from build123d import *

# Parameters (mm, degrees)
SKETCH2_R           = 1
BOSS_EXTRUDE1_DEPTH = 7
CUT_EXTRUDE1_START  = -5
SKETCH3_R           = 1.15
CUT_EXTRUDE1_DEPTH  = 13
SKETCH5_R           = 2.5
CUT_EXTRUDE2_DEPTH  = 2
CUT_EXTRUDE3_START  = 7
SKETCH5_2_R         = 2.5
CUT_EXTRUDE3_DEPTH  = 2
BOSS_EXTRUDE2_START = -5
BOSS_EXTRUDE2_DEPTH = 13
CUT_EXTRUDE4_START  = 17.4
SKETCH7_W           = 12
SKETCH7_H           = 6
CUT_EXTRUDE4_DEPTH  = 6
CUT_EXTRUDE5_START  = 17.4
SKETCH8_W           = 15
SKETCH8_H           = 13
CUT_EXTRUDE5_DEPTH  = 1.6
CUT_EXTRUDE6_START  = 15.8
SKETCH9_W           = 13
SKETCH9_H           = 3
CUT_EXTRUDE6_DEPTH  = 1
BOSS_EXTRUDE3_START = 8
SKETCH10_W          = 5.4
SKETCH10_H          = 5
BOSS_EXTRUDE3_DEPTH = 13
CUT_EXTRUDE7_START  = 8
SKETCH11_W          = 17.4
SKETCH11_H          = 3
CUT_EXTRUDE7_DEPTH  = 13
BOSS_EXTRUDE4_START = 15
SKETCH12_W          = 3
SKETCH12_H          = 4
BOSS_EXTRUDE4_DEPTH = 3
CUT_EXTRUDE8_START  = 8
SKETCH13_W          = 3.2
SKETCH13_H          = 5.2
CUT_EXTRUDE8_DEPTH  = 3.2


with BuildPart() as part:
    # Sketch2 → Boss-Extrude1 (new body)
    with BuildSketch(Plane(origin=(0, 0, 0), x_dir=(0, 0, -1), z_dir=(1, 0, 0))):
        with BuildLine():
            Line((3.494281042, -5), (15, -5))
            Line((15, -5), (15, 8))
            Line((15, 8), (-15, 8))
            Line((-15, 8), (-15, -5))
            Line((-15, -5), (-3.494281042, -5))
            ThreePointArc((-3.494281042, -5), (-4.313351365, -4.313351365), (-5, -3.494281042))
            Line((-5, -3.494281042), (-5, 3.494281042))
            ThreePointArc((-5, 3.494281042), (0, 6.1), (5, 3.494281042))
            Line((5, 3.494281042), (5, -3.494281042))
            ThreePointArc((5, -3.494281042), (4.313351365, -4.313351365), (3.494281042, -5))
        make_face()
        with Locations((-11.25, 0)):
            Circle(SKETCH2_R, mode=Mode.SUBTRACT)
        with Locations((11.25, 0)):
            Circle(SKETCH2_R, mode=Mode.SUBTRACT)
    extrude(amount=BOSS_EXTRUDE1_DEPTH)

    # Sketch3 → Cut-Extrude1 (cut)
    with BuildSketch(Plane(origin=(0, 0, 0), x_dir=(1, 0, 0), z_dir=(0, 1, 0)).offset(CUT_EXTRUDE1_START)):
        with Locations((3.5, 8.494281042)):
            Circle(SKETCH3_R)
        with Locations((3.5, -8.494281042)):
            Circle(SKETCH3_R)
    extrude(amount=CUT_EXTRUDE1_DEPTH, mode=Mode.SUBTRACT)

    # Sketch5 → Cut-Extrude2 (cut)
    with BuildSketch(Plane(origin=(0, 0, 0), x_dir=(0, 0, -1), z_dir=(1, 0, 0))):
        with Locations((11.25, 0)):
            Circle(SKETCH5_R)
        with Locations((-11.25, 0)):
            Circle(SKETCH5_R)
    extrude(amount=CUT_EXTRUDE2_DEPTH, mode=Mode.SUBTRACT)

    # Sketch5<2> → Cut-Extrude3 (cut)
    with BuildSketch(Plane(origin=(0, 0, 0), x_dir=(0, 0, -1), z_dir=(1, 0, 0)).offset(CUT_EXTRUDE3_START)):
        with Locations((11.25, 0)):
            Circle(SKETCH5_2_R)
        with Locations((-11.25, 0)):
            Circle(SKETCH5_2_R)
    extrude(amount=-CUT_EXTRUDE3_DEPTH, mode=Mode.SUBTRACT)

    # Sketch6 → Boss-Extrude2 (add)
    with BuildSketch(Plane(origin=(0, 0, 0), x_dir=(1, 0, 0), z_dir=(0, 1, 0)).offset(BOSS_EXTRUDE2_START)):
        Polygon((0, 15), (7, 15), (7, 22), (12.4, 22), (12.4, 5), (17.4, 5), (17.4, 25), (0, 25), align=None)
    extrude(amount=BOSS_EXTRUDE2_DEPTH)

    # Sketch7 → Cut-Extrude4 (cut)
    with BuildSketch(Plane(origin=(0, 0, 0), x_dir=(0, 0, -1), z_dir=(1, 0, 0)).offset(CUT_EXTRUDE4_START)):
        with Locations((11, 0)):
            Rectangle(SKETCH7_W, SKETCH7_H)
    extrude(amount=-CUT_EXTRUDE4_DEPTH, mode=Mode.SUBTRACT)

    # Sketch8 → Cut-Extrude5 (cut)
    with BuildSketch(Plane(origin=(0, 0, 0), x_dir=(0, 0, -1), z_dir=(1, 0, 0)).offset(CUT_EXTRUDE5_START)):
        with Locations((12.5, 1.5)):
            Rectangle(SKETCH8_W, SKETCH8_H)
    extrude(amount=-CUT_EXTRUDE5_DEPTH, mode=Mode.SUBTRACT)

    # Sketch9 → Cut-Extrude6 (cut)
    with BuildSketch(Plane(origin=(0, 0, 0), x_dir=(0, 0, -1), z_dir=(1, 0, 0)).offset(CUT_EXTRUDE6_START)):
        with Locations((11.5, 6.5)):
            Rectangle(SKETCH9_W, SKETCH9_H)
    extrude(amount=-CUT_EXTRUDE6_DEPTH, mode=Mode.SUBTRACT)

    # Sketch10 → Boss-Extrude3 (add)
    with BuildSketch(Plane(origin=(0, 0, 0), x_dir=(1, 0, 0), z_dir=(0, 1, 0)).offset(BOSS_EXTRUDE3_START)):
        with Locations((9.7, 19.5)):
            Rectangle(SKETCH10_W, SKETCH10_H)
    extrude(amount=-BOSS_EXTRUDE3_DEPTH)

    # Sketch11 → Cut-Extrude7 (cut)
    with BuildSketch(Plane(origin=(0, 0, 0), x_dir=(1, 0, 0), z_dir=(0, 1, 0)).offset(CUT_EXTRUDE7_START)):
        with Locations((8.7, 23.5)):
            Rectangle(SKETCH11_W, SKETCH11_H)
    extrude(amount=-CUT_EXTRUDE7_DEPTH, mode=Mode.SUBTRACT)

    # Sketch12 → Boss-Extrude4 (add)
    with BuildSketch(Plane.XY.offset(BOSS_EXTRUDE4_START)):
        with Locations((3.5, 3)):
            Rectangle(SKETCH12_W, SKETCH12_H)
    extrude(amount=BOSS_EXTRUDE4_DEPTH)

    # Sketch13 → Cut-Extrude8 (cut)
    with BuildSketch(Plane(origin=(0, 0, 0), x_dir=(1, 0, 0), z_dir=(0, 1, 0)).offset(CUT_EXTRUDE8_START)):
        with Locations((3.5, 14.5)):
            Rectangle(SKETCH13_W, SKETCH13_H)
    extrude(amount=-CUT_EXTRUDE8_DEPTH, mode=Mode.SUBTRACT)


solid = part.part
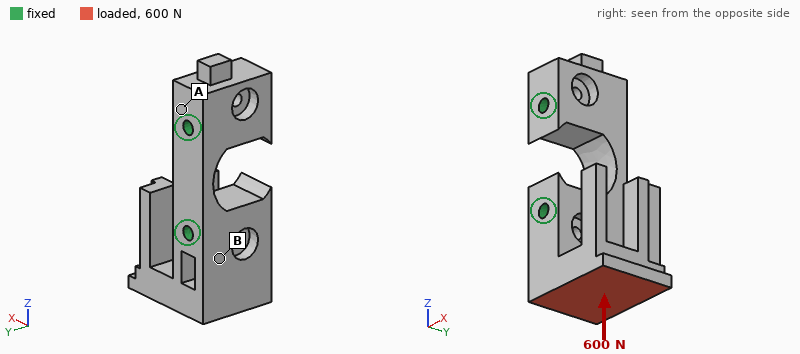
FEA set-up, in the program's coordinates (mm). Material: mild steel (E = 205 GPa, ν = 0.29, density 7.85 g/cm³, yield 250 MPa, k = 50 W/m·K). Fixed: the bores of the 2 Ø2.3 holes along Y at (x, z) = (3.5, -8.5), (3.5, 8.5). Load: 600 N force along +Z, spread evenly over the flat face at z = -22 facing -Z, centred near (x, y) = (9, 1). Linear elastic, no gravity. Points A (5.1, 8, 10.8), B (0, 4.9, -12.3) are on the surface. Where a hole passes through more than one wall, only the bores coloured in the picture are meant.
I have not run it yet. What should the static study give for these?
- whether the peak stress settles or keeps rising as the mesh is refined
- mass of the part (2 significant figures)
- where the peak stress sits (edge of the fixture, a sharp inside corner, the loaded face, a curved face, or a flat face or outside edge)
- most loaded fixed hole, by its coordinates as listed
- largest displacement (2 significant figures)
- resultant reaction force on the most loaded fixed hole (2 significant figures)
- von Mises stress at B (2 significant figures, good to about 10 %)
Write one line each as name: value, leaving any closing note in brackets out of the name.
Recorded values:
whether the peak stress settles or keeps rising as the mesh is refined: keeps rising
mass of the part: 25 g
where the peak stress sits: edge of the fixture
most loaded fixed hole, by its coordinates as listed: (3.5, -8.5)
largest displacement: 16 µm
resultant reaction force on the most loaded fixed hole: 590 N
von Mises stress at B: 36 MPa
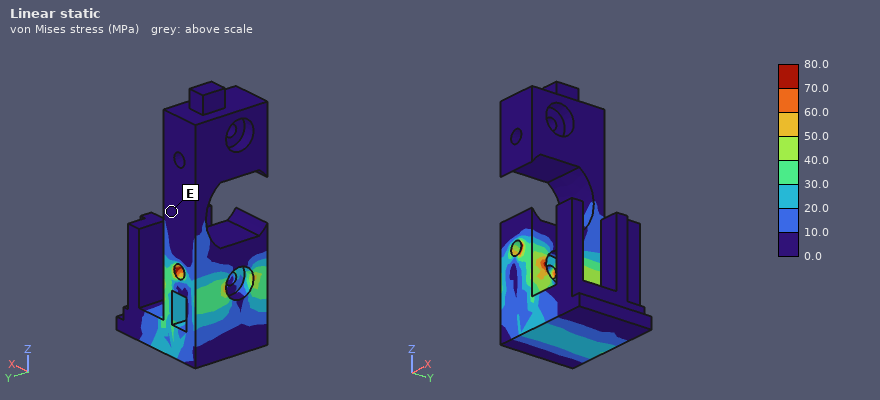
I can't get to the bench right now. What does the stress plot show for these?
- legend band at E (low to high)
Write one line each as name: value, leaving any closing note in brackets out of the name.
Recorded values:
legend band at E: 0.0 to 10.0 MPa
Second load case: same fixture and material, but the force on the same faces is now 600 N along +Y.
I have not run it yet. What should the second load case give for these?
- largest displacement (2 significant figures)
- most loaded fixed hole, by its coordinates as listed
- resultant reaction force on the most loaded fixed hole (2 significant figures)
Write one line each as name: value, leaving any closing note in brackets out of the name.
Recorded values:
largest displacement: 13 µm
most loaded fixed hole, by its coordinates as listed: (3.5, -8.5)
resultant reaction force on the most loaded fixed hole: 600 N
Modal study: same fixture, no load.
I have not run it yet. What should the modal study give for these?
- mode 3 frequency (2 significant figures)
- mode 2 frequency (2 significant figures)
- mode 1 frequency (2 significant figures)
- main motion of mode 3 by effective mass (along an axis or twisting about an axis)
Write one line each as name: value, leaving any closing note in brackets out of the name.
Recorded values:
mode 3 frequency: 12 kHz
mode 2 frequency: 9100 Hz
mode 1 frequency: 9000 Hz
main motion of mode 3 by effective mass: along X
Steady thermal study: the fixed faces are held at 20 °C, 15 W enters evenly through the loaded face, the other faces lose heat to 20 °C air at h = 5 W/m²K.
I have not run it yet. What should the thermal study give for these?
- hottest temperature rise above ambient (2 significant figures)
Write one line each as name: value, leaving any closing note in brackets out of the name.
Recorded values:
hottest temperature rise above ambient: 63 K
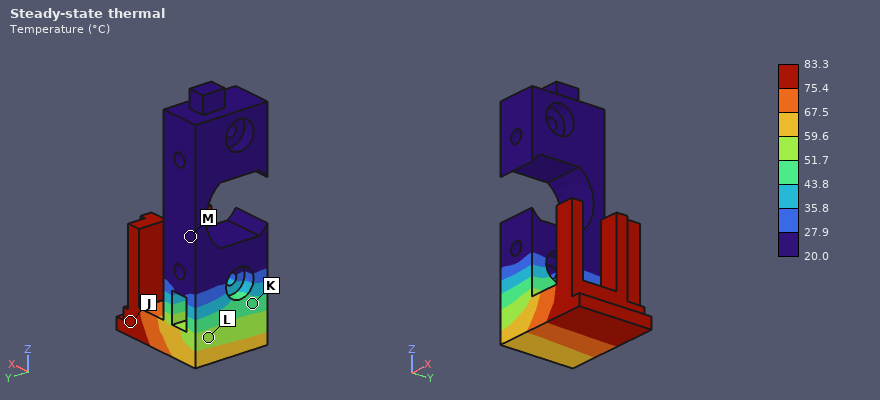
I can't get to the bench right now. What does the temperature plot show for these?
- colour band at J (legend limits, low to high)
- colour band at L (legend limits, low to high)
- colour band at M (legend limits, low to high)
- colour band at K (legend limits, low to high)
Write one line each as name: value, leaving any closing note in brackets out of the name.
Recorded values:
colour band at J: 75.4 to 83.3 °C
colour band at L: 51.7 to 59.6 °C
colour band at M: 20.0 to 27.9 °C
colour band at K: 43.8 to 51.7 °C
